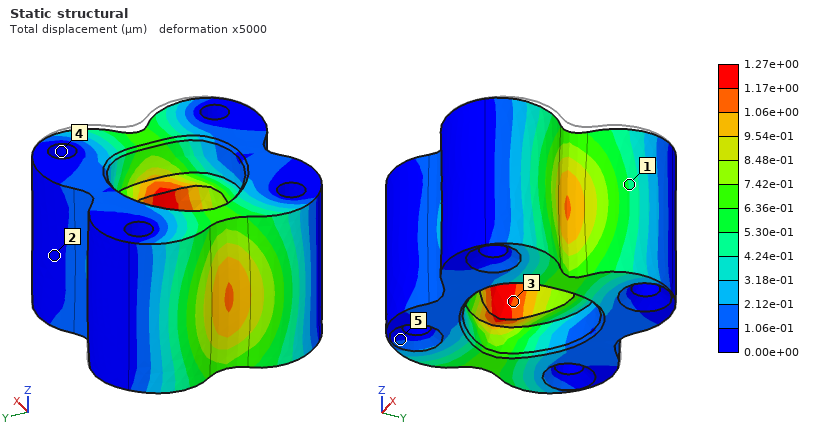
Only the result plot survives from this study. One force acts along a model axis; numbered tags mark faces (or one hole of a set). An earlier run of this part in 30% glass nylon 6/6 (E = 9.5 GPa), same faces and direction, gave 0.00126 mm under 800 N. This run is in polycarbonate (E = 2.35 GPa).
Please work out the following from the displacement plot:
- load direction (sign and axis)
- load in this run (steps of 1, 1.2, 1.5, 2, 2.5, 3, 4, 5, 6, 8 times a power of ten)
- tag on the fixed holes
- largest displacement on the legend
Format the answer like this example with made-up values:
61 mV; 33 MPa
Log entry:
-X; 200 N; 4; 1.27e+00 µm
